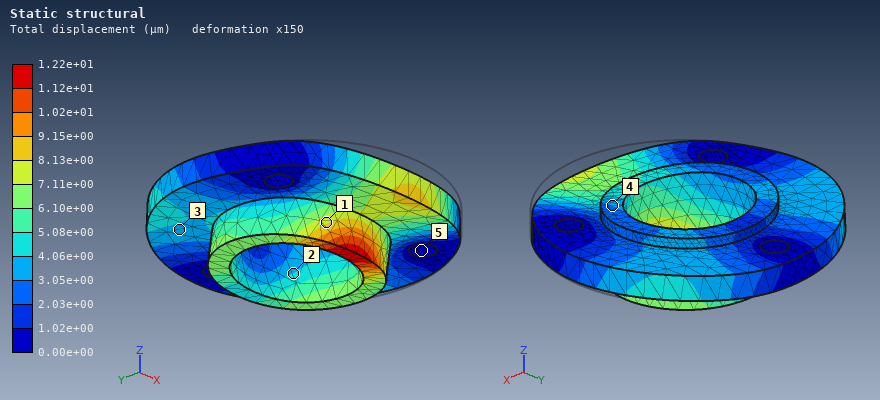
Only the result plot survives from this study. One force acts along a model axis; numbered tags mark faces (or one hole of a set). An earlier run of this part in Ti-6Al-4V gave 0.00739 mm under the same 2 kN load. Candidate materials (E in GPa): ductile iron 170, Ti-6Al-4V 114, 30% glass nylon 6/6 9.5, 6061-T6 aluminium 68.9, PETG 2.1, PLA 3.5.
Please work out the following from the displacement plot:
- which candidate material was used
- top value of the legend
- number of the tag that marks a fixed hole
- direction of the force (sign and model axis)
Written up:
6061-T6 aluminium
1.22e+01 µm
5
+Y
